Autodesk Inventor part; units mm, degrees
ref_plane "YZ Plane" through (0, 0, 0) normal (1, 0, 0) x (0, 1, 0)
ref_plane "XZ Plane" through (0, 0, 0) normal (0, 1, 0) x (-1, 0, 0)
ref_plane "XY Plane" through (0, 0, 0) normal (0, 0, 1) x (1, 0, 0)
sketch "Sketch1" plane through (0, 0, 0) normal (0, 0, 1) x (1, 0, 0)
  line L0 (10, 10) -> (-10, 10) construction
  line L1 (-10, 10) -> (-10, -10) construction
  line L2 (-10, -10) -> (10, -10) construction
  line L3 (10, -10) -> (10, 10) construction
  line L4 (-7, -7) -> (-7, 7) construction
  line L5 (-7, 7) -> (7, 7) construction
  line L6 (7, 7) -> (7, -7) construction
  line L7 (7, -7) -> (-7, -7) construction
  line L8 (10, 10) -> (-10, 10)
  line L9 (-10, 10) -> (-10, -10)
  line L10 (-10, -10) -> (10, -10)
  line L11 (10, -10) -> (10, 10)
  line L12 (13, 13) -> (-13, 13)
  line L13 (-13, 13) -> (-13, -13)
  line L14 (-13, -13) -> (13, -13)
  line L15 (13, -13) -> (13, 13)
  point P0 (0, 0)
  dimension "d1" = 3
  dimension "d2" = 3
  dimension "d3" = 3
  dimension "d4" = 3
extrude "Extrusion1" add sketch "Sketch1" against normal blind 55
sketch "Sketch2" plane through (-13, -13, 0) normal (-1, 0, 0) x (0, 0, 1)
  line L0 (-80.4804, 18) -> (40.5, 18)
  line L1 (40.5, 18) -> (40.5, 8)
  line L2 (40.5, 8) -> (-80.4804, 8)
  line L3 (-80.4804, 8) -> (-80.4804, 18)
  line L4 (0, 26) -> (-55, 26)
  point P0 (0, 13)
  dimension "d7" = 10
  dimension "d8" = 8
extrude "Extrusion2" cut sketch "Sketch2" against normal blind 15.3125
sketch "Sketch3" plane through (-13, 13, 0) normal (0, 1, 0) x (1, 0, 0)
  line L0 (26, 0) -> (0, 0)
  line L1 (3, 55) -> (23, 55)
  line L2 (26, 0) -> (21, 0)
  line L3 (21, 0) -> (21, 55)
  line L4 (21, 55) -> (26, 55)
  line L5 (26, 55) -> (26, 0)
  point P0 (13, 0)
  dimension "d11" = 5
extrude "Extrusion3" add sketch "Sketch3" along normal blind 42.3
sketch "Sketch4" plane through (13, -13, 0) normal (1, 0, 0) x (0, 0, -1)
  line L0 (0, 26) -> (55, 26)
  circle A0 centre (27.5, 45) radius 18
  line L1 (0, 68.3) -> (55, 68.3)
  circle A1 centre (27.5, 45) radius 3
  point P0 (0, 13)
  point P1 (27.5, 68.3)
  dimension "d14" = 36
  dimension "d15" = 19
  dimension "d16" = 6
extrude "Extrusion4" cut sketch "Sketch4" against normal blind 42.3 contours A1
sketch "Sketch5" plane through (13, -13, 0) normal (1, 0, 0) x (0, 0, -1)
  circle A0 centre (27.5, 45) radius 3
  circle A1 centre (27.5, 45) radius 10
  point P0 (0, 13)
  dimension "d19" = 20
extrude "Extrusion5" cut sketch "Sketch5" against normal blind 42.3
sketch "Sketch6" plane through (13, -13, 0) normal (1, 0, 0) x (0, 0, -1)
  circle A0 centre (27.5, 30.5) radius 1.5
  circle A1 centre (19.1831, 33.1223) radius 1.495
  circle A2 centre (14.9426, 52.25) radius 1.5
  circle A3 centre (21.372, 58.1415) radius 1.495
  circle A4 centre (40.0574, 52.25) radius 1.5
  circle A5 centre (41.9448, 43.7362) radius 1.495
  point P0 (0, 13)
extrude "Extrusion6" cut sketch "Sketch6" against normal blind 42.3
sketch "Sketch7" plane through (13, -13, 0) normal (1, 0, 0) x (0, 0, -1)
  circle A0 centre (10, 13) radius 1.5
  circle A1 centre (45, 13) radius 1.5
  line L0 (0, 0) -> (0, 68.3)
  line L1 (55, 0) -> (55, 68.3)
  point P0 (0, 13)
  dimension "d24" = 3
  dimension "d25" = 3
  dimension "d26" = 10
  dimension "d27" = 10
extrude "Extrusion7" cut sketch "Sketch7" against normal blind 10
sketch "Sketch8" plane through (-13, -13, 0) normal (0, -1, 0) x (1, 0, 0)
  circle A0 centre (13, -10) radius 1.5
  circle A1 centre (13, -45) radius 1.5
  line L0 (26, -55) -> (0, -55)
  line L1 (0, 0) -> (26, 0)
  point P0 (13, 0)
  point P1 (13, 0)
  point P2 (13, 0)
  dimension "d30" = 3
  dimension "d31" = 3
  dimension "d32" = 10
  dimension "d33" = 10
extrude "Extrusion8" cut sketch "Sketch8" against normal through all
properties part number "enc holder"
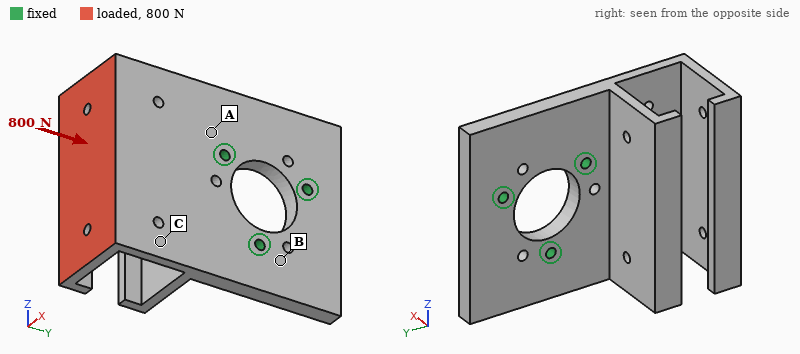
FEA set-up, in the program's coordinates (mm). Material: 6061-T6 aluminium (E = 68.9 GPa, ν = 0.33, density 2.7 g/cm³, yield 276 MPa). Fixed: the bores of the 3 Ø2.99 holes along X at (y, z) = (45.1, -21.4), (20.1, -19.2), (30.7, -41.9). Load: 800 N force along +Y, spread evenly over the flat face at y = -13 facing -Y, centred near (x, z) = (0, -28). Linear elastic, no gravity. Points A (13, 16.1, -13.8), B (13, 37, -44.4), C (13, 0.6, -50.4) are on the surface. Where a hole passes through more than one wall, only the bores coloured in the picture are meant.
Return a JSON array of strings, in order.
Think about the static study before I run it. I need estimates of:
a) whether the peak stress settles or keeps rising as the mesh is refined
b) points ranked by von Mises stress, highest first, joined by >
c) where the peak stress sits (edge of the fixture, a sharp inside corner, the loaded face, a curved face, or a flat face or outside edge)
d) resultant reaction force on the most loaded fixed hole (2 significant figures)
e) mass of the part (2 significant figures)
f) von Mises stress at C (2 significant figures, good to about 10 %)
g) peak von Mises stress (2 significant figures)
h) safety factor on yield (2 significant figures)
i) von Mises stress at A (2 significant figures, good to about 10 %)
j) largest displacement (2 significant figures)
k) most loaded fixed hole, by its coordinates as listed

["settles", "C > A > B", "a curved face", "430 N", "63 g", "110 MPa", "240 MPa", "1.2", "37 MPa", "0.87 mm", "(20.1, -19.2)"]
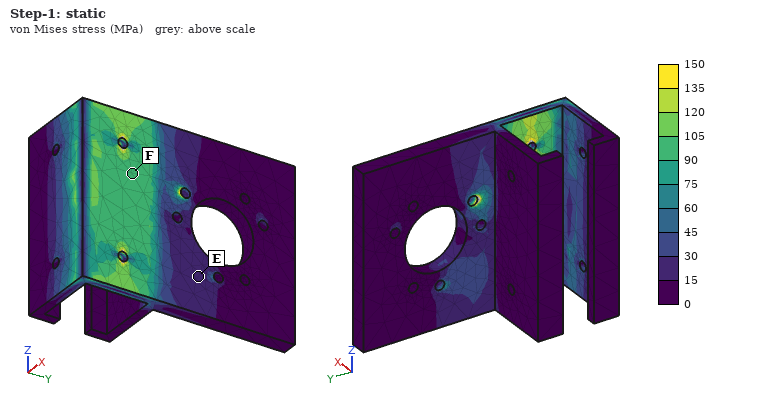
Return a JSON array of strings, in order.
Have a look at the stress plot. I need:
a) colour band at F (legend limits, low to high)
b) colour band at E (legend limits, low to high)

["90 to 105 MPa", "15 to 30 MPa"]
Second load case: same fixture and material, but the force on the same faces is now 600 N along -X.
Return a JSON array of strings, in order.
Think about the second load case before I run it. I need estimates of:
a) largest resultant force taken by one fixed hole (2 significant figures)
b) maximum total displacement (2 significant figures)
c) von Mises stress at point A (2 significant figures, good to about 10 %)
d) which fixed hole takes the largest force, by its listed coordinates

["790 N", "0.89 mm", "85 MPa", "(20.1, -19.2)"]
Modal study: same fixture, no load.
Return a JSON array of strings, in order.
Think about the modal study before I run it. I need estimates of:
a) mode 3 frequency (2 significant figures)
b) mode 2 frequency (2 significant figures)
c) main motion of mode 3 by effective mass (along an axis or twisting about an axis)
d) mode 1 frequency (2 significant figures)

["2500 Hz", "1700 Hz", "along X", "1100 Hz"]
